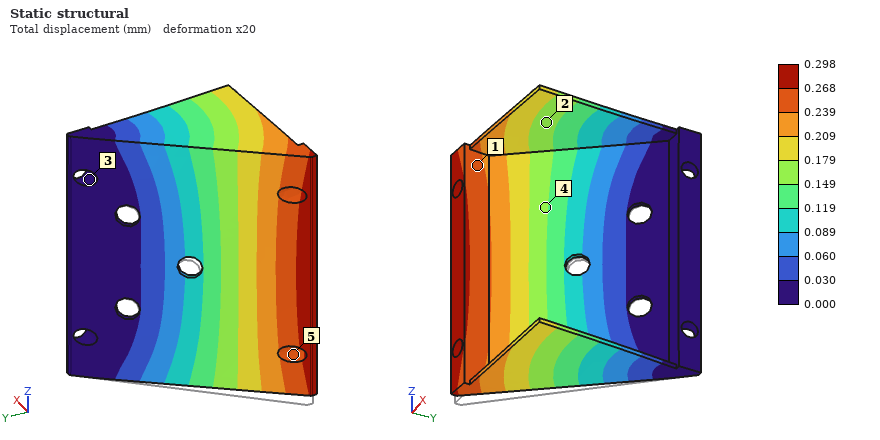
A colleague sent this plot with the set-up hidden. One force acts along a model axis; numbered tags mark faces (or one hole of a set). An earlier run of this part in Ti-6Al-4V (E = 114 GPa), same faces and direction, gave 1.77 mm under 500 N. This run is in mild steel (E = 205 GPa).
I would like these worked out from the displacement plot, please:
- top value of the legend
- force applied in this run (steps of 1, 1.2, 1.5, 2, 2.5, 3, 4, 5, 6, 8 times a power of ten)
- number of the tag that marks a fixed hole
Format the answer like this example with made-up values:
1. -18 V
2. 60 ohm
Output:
1. 0.298 mm
2. 150 N
3. 3
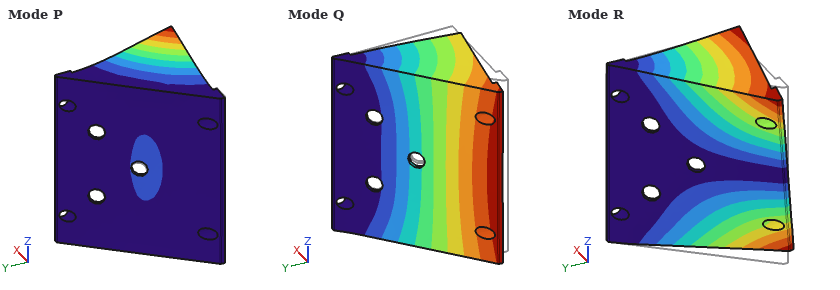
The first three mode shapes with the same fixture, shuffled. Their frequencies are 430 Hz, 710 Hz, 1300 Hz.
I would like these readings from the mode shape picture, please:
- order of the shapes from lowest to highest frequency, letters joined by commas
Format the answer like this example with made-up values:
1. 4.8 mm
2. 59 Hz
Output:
1. Q, R, P
